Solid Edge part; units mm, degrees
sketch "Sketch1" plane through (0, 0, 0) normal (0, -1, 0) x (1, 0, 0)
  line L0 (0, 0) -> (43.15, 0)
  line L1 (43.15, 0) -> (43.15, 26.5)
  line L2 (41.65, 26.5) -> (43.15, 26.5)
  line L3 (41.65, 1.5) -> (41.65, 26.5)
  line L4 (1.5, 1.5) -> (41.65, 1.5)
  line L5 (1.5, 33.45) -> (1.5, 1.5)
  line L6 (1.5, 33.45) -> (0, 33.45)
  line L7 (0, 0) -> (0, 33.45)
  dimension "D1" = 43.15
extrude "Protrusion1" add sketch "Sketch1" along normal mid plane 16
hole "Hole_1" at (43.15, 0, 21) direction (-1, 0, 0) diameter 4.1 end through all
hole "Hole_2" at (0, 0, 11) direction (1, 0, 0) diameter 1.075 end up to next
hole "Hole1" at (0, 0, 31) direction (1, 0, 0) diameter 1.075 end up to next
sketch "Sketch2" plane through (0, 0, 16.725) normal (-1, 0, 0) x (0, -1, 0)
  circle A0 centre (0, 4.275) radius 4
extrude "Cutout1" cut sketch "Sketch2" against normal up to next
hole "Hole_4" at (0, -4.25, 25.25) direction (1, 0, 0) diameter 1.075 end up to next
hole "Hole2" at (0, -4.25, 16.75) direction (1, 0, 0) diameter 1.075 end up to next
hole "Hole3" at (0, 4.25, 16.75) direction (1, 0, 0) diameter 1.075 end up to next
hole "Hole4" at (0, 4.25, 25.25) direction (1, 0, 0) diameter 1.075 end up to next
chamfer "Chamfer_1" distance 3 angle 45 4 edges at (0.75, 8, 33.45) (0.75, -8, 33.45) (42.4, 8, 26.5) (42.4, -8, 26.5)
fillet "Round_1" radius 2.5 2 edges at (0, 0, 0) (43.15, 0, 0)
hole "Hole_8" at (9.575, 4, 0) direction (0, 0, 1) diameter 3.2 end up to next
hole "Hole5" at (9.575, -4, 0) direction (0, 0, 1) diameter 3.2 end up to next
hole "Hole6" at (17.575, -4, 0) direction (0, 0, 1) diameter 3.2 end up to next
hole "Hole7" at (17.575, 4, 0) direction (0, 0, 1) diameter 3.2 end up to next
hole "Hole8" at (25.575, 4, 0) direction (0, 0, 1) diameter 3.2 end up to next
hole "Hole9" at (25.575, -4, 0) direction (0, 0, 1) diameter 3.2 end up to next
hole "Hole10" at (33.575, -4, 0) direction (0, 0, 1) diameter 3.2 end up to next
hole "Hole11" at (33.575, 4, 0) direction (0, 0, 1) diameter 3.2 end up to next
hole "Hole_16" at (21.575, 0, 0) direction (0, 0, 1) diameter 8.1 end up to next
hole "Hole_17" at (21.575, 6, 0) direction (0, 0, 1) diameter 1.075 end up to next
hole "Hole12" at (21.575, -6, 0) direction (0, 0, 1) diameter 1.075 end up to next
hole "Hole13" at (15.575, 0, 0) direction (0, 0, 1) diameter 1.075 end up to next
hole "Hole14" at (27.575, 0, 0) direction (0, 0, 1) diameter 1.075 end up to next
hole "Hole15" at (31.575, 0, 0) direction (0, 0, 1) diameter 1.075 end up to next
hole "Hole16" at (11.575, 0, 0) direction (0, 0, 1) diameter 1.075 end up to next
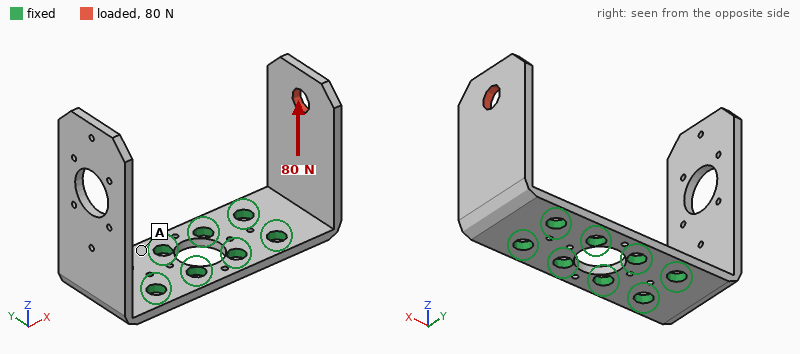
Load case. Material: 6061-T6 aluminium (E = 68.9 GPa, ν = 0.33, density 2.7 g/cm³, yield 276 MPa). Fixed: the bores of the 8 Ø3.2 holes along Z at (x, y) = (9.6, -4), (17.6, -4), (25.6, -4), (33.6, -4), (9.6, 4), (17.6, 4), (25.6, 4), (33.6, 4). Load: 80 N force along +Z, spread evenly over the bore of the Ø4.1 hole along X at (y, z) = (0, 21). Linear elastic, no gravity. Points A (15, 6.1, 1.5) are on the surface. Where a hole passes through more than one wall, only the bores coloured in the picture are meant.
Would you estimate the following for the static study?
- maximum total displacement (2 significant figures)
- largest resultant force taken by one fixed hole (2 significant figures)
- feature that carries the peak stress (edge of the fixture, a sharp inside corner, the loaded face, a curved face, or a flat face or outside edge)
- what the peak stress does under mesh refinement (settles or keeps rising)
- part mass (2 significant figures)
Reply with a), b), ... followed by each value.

a) 0.20 mm
b) 41 N
c) edge of the fixture
d) keeps rising
e) 5.5 g
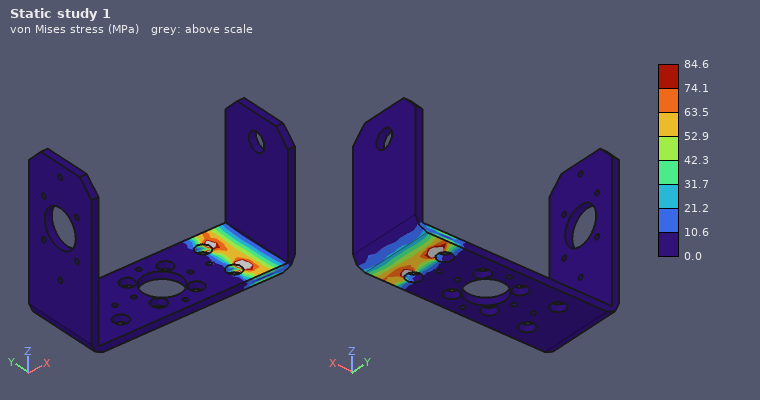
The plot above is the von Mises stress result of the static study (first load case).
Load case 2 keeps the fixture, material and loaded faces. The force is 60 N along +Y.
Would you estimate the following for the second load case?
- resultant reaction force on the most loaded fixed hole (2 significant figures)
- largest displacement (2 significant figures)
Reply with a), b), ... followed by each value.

a) 130 N
b) 0.25 mm
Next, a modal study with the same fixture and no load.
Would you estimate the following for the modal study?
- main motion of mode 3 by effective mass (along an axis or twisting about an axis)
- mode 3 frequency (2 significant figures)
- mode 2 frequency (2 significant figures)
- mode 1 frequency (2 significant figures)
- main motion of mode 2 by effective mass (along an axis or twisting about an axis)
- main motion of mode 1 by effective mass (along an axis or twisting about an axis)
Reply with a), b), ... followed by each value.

a) along Y
b) 2200 Hz
c) 1400 Hz
d) 910 Hz
e) along X
f) along X
